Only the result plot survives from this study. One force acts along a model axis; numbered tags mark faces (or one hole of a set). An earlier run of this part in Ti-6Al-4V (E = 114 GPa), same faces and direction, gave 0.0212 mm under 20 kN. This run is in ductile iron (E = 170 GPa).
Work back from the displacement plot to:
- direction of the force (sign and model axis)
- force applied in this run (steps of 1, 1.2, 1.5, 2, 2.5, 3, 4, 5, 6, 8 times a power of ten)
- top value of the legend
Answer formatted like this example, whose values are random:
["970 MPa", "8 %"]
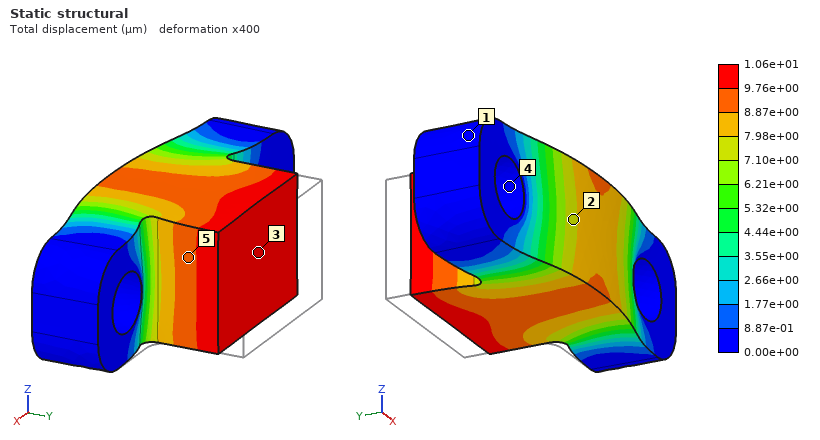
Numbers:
["-Y", "15 kN", "1.06e+01 µm"]
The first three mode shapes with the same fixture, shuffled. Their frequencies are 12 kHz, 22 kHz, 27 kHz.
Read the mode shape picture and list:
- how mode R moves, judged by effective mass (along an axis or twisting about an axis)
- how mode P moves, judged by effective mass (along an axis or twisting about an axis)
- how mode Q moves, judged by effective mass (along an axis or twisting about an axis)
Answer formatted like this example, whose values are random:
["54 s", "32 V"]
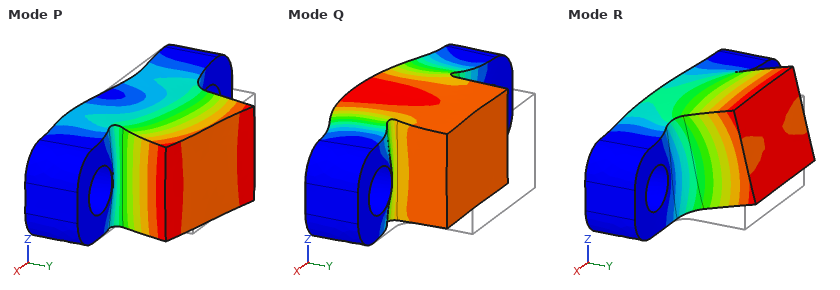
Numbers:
["along Z", "along X", "along Y"]
